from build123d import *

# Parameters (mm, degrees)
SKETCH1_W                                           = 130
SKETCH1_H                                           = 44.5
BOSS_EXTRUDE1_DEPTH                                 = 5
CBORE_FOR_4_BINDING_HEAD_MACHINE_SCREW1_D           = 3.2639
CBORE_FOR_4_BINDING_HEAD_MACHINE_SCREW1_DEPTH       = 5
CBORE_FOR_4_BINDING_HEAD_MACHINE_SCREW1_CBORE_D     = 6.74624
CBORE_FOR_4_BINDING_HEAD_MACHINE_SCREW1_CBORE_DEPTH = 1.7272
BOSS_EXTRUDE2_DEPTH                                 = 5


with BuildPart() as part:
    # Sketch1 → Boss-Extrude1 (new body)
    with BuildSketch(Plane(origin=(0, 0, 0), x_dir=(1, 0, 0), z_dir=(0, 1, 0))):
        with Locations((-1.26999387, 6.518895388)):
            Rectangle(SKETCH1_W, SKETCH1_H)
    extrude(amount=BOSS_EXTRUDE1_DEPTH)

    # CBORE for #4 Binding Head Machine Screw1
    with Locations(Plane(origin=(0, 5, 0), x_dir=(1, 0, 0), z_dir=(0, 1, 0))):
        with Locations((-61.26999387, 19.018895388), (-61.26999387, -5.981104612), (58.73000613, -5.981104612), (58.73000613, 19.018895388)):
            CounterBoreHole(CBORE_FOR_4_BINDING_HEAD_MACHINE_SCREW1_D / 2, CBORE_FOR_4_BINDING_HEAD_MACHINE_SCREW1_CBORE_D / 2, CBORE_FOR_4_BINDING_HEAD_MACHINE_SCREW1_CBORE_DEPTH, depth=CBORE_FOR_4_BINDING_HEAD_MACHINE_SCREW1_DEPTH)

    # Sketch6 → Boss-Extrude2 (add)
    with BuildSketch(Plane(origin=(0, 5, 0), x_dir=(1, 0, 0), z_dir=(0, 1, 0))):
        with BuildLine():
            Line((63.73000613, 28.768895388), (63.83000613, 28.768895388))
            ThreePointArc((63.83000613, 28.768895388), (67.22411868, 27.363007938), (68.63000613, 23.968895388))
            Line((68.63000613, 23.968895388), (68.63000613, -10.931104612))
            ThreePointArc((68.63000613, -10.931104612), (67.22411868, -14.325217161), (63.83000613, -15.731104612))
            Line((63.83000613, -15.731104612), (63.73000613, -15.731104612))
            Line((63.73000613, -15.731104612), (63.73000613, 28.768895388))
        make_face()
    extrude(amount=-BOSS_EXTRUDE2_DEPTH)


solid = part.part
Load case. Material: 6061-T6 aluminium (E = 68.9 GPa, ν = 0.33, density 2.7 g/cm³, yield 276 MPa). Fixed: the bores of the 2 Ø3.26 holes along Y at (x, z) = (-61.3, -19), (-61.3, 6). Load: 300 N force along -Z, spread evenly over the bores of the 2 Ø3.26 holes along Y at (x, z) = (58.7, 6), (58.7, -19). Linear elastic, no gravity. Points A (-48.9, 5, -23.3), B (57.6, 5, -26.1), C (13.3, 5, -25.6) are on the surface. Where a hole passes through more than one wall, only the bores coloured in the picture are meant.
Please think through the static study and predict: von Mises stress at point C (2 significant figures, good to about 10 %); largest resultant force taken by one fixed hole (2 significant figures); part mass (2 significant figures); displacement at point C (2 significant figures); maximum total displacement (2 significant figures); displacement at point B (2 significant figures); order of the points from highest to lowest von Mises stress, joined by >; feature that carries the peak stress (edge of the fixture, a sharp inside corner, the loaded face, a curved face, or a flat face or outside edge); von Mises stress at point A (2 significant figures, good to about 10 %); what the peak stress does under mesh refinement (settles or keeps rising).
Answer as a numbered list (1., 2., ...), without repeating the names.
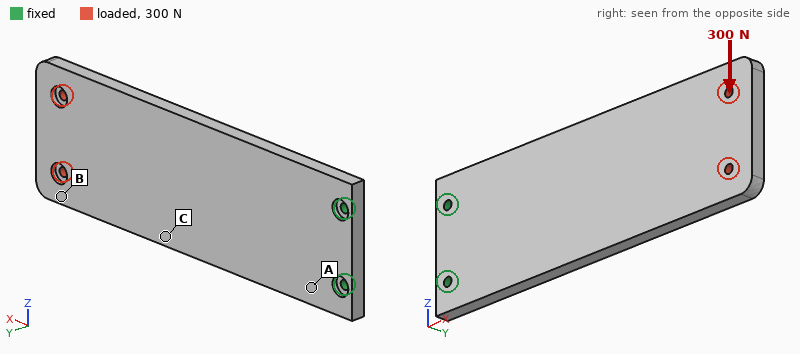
1. 7.1 MPa
2. 1.4 kN
3. 80 g
4. 0.057 mm
5. 0.12 mm
6. 0.10 mm
7. A > C > B
8. edge of the fixture
9. 13 MPa
10. keeps rising
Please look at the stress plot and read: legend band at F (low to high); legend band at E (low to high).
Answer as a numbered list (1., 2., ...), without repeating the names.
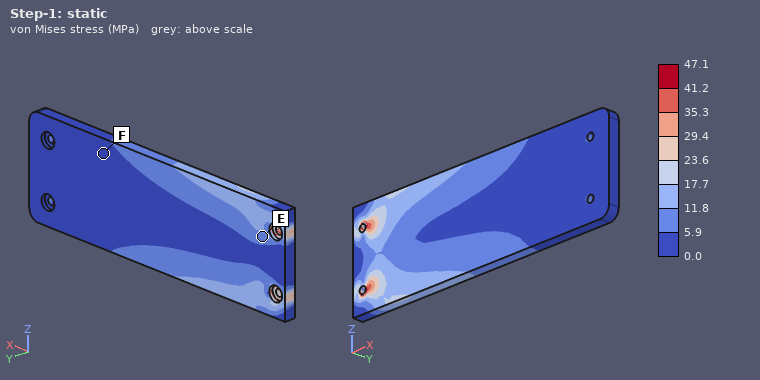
1. 0.0 to 5.9 MPa
2. 5.9 to 11.8 MPa
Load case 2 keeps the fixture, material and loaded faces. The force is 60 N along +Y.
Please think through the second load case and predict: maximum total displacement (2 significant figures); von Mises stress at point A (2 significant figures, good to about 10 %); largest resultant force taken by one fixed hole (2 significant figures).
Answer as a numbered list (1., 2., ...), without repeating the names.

1. 1.4 mm
2. 35 MPa
3. 52 N
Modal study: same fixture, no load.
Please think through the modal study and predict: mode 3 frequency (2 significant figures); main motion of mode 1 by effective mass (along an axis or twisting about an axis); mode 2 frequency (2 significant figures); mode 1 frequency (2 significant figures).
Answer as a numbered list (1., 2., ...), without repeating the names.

1. 1400 Hz
2. along Y
3. 1400 Hz
4. 220 Hz
